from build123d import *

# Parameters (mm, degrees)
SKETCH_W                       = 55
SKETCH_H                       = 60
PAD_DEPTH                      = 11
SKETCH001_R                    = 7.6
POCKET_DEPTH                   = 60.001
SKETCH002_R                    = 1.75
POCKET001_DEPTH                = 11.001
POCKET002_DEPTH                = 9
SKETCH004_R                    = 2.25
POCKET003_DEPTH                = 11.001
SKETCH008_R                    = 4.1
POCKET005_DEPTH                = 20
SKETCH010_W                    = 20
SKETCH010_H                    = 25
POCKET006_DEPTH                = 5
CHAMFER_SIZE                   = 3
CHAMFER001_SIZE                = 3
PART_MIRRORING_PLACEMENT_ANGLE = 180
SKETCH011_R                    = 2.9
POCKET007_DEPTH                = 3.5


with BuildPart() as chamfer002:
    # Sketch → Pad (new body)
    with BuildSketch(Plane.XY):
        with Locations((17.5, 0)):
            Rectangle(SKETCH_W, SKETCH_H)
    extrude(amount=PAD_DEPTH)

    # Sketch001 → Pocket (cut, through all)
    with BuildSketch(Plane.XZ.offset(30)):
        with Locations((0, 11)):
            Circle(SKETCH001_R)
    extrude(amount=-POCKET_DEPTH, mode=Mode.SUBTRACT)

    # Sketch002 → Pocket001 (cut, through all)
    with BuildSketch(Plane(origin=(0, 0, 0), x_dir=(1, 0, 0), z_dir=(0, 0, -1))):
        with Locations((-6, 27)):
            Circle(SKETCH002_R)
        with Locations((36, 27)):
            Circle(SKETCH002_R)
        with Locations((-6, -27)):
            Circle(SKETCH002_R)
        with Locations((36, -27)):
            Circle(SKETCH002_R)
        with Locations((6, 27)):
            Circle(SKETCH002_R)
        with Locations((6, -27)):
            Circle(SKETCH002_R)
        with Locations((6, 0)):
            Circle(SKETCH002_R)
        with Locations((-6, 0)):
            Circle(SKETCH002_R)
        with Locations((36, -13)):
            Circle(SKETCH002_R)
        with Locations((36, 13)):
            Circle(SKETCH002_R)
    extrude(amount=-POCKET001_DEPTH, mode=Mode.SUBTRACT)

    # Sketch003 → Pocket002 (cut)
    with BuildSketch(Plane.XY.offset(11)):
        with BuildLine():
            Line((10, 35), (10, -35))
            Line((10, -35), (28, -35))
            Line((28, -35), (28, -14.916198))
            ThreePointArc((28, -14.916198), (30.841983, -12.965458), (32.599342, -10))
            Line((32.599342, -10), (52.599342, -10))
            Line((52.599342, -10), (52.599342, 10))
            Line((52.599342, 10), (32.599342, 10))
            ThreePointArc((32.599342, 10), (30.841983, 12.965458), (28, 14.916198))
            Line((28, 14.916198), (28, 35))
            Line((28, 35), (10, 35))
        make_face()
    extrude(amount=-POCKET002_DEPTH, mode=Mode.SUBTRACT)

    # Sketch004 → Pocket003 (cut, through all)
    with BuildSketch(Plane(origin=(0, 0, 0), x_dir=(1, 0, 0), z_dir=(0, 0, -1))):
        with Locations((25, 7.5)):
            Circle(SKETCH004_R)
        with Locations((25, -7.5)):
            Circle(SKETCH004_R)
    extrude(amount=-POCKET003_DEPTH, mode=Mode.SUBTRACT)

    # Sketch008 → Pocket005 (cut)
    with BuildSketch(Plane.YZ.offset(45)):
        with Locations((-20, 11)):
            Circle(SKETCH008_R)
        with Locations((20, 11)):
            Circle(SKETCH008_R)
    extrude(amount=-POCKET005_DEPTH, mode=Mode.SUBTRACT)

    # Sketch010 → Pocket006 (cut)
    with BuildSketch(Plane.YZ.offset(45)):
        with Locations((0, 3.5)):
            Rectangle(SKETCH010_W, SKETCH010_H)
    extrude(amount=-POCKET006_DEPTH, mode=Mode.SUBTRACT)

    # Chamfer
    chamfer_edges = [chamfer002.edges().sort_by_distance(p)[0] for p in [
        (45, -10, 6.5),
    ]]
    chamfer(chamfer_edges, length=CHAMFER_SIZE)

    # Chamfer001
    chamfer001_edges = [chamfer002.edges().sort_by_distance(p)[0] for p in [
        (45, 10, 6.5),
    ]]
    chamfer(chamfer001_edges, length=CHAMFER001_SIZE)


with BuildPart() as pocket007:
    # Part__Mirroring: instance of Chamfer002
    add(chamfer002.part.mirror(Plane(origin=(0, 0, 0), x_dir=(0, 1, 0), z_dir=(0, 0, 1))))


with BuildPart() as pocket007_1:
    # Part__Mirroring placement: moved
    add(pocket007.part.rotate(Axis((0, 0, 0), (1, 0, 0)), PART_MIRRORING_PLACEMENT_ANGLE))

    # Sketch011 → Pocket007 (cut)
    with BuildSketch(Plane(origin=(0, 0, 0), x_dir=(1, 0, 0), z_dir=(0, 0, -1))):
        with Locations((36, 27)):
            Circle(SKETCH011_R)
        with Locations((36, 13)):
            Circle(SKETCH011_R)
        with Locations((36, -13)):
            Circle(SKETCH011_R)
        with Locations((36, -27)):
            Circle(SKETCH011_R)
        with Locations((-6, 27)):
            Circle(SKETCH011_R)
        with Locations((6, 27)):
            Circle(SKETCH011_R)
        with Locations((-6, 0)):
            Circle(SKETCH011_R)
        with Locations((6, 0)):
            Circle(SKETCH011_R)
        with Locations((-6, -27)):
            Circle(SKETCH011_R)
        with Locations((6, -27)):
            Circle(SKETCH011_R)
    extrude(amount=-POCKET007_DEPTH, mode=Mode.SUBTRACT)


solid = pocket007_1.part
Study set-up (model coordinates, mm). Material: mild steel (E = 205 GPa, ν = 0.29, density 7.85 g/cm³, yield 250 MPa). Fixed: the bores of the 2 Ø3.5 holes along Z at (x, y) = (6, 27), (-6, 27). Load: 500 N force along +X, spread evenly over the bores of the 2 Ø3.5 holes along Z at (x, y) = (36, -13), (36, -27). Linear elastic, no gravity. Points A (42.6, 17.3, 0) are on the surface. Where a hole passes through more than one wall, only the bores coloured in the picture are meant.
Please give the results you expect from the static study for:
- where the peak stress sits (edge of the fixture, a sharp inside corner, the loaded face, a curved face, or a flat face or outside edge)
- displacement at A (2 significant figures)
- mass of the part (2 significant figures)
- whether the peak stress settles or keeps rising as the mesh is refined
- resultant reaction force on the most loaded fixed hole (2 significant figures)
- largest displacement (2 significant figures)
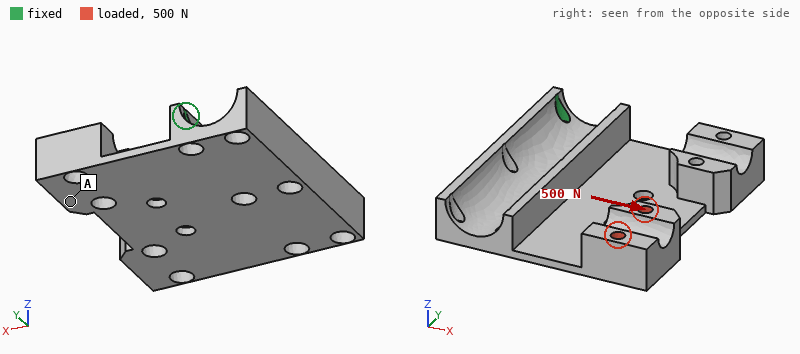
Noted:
edge of the fixture
0.16 mm
120 g
keeps rising
1.4 kN
0.38 mm
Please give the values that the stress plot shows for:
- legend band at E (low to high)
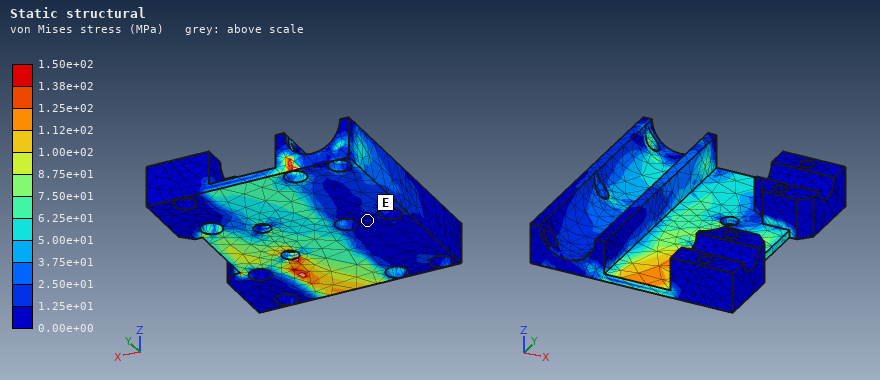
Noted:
0.00e+00 to 1.25e+01 MPa
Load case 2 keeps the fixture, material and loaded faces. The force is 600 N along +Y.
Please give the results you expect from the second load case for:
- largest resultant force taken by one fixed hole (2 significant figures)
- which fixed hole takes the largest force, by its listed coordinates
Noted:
1.7 kN
(6, 27)
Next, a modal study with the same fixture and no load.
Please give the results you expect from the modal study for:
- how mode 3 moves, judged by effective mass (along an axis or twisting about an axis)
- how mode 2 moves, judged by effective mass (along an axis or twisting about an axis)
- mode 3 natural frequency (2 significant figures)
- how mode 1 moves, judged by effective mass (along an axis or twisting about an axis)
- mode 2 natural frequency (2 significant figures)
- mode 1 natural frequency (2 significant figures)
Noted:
along Z
twisting about X
2000 Hz
along Z
1100 Hz
620 Hz
